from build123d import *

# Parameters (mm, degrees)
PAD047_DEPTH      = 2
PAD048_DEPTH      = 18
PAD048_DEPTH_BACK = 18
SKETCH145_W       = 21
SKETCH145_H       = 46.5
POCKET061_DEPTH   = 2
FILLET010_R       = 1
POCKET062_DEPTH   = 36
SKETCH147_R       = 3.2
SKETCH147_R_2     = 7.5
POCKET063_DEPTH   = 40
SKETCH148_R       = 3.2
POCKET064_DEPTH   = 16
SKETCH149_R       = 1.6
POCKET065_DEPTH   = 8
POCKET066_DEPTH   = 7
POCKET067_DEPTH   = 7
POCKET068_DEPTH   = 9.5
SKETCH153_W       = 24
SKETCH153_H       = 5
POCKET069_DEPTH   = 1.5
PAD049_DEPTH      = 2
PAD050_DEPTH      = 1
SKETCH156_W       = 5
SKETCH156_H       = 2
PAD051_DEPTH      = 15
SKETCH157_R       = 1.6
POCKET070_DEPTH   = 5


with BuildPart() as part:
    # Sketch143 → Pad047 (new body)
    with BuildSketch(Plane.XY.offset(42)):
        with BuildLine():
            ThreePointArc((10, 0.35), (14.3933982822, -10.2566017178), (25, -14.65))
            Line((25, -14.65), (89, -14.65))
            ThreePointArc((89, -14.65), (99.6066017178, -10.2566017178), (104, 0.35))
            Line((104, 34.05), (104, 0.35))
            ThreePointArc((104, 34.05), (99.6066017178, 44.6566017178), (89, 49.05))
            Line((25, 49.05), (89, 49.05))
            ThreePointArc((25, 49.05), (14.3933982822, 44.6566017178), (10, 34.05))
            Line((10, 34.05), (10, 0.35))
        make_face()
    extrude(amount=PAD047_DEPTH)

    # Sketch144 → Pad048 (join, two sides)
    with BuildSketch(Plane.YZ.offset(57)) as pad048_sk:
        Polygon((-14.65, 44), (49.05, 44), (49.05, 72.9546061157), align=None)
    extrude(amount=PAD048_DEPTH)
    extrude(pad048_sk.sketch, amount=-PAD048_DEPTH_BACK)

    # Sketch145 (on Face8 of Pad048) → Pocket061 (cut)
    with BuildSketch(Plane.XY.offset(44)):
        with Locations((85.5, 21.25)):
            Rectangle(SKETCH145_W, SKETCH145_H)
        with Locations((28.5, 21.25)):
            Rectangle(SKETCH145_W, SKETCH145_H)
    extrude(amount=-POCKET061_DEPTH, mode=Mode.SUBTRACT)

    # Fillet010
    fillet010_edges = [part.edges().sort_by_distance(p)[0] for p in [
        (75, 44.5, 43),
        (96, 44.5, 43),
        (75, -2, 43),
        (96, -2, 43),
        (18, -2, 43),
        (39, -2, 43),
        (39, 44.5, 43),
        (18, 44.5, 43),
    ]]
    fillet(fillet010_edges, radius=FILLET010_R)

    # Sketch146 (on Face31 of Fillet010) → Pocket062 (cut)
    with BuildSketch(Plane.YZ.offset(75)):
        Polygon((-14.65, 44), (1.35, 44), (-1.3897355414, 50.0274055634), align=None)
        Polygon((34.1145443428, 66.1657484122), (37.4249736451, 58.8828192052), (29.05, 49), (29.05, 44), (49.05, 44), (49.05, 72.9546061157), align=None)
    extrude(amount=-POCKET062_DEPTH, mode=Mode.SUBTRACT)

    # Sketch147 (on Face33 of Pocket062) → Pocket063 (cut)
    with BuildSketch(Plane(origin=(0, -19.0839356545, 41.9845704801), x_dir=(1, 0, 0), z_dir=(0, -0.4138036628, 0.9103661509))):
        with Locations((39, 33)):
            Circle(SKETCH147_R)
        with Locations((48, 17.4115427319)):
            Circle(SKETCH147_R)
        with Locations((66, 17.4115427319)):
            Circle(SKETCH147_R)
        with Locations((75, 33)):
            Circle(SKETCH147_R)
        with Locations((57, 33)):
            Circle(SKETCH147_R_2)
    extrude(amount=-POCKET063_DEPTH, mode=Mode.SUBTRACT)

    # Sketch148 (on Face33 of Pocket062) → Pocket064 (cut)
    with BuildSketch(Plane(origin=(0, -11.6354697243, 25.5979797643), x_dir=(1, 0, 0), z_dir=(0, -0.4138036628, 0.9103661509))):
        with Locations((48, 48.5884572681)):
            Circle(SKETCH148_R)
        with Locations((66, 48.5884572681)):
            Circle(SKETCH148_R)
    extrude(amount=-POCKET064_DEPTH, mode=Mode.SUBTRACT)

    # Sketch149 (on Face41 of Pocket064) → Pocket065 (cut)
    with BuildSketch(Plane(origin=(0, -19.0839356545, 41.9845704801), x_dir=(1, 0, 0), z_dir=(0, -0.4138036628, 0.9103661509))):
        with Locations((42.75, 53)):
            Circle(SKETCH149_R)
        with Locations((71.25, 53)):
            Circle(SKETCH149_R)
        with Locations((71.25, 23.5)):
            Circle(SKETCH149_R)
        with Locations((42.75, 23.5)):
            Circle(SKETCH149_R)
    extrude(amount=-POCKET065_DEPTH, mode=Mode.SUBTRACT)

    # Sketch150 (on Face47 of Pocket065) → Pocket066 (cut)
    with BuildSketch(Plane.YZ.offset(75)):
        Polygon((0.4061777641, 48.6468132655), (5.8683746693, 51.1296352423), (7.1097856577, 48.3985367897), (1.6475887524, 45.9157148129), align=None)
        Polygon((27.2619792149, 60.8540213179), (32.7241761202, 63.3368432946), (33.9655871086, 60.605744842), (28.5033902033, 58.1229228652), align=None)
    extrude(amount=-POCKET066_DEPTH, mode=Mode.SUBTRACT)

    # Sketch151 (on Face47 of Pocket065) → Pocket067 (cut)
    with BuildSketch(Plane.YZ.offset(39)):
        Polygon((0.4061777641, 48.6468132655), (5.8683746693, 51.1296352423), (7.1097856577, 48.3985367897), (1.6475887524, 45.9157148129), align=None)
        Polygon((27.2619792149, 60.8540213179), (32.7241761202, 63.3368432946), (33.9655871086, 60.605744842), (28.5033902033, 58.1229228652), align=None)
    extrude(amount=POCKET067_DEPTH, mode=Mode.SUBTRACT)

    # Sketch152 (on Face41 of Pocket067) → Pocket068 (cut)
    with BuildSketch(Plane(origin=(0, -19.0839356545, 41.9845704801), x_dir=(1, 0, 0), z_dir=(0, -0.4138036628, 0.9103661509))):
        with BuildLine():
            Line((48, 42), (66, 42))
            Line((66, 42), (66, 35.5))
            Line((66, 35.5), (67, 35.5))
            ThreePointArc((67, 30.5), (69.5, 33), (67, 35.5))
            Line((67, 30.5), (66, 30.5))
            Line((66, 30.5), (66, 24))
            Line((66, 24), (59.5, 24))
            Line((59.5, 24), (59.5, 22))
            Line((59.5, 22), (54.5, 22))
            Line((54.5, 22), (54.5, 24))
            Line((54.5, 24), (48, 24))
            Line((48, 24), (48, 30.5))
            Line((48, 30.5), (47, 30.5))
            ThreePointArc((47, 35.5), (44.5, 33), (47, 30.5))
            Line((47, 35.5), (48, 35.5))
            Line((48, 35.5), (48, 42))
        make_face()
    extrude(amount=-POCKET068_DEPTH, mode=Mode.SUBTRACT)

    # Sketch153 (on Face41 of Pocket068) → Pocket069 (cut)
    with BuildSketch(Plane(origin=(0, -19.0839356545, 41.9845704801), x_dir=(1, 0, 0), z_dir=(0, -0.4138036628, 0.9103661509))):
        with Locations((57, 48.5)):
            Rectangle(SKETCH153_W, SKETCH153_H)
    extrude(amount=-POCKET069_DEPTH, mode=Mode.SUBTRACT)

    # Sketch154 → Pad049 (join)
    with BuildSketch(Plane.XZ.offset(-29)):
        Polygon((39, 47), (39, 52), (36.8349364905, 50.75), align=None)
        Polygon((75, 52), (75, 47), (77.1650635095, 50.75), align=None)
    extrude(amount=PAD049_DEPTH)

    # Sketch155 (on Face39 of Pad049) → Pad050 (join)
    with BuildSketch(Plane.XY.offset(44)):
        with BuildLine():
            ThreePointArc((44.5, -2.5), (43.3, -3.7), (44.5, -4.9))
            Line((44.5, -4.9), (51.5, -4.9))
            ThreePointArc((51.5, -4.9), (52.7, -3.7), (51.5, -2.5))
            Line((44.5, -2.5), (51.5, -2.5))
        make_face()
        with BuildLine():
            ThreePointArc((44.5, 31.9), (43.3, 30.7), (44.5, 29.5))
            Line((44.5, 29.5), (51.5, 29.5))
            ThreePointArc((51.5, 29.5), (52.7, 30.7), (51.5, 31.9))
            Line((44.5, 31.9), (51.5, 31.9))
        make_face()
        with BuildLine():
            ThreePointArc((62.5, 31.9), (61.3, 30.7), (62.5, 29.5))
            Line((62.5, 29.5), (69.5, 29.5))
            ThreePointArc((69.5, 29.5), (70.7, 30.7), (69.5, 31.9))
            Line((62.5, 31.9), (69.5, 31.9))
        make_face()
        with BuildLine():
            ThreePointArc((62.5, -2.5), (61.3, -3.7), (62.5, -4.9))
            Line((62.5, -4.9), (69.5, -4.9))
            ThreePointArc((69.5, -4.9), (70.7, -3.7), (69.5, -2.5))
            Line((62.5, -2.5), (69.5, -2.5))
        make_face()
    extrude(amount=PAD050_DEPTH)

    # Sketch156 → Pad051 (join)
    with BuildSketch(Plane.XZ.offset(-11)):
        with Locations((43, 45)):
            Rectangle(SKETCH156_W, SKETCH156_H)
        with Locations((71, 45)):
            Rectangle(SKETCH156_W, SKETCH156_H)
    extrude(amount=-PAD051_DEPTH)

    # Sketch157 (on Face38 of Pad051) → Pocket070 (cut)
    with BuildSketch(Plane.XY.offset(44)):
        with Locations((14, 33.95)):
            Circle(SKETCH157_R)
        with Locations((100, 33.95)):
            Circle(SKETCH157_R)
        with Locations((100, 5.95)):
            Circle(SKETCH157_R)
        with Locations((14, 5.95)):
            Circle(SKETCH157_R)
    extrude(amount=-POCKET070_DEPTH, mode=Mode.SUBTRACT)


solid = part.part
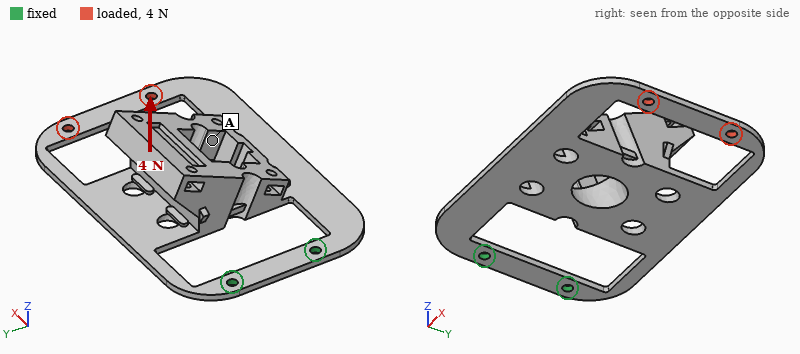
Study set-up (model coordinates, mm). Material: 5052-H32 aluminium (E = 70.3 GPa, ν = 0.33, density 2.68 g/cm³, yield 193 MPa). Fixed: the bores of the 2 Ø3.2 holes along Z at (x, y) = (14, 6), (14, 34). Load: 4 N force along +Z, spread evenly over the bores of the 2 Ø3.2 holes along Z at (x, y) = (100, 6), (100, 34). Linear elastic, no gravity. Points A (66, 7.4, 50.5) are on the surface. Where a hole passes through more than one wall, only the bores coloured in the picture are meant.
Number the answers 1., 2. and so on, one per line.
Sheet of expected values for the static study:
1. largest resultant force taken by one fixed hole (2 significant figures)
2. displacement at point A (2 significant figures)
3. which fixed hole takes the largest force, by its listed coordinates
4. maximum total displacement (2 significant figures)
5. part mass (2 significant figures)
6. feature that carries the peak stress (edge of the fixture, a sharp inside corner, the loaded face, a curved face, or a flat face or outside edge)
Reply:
1. 2.1 N
2. 0.63 mm
3. (14, 6)
4. 1.3 mm
5. 50 g
6. a flat face or outside edge
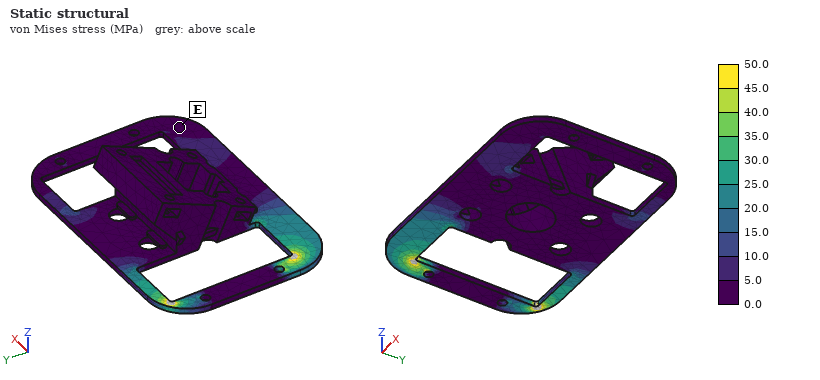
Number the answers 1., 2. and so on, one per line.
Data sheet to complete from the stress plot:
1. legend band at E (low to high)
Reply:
1. 0.0 to 5.0 MPa
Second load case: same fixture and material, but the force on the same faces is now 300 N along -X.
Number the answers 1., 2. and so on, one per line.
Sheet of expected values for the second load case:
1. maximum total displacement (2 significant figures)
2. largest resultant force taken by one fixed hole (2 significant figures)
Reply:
1. 88 µm
2. 160 N
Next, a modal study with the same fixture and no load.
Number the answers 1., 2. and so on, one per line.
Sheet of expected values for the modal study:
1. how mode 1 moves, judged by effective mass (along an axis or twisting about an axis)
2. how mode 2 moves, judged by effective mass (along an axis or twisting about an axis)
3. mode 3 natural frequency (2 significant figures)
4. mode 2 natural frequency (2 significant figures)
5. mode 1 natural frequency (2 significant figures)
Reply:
1. along Z
2. along Y
3. 660 Hz
4. 390 Hz
5. 83 Hz
